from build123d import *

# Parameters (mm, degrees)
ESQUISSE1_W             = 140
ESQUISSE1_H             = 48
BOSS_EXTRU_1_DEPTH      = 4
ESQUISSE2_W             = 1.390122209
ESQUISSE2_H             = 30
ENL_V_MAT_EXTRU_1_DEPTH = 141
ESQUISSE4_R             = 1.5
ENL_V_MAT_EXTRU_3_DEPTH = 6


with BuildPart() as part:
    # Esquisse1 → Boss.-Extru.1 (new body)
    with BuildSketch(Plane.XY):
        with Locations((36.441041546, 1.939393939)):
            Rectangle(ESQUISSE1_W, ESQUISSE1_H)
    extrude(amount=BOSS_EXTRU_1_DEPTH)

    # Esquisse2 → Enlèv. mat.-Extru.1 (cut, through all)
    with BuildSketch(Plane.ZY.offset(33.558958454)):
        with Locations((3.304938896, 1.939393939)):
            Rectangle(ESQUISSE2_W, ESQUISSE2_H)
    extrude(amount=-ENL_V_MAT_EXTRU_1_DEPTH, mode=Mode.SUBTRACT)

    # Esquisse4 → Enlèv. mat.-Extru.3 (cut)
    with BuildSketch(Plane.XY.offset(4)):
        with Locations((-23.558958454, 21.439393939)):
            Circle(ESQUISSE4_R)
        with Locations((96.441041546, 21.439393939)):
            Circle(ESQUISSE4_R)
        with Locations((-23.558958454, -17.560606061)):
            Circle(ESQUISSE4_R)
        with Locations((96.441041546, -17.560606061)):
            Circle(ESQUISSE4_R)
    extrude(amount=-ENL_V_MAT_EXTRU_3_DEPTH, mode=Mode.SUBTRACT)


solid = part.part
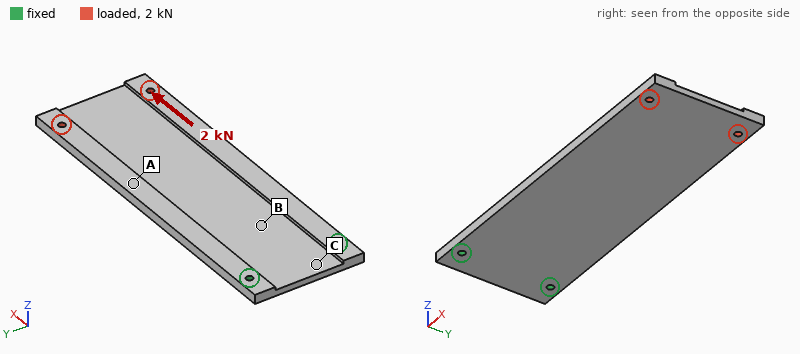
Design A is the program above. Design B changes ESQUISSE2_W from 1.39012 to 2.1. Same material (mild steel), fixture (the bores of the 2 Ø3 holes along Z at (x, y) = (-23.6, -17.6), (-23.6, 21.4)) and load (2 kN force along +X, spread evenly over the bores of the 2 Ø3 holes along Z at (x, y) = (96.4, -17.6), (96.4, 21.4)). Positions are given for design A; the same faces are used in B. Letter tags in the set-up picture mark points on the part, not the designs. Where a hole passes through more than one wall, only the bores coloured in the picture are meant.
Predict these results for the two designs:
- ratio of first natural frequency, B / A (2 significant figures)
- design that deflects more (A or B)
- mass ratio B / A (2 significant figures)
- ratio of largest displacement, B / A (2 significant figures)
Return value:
1.0
B
0.93
1.2
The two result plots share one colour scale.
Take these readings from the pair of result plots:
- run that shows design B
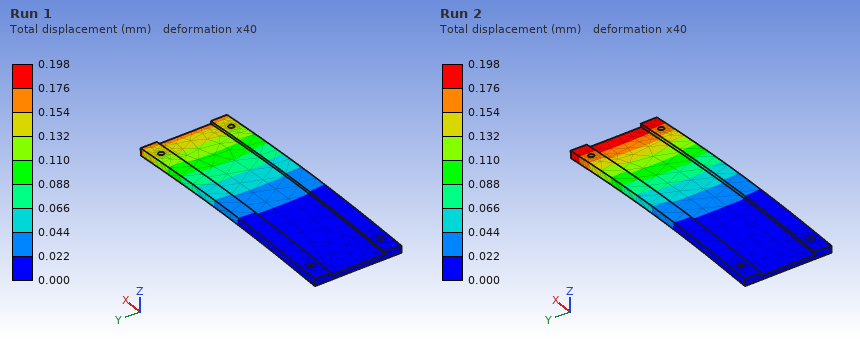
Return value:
Run 2
